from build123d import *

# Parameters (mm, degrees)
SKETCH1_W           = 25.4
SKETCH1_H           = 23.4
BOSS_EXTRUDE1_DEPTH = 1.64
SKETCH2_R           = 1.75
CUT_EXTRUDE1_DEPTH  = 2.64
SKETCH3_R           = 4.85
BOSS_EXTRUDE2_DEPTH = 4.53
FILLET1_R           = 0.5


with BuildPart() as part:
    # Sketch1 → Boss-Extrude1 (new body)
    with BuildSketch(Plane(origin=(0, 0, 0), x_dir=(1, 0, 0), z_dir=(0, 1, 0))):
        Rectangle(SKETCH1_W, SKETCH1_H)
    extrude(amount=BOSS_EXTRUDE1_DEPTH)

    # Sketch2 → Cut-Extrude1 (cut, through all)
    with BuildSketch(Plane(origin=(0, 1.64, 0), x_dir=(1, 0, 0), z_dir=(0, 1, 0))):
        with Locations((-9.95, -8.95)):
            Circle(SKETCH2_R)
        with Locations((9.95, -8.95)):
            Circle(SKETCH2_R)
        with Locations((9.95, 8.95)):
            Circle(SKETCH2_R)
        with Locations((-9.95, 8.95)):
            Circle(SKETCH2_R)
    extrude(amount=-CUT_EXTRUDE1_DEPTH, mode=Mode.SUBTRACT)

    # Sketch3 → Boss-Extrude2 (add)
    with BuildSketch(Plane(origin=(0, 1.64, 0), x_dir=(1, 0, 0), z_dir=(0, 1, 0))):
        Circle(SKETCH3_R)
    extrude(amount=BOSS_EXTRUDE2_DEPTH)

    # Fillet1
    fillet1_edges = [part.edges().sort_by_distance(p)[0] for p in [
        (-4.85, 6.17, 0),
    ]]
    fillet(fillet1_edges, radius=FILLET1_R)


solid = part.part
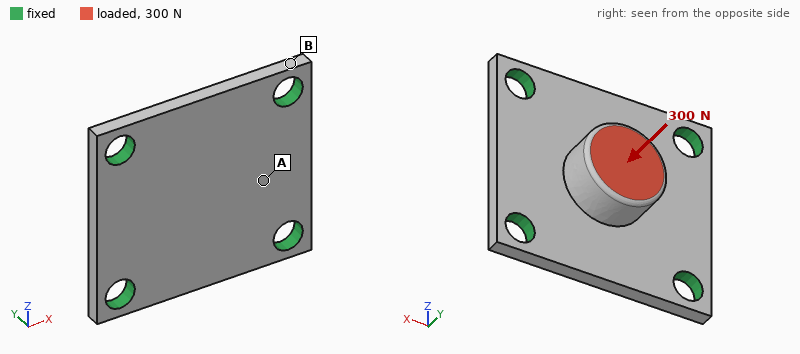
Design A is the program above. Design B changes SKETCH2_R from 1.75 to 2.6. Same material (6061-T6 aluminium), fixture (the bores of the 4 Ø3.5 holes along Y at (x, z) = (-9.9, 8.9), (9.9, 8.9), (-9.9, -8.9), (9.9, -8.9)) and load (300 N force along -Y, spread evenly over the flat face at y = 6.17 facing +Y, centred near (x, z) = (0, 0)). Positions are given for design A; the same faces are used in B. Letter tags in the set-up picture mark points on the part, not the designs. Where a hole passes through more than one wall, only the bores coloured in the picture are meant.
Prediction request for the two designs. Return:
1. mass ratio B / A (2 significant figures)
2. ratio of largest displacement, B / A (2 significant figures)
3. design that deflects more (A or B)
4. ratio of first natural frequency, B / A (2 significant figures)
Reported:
0.94
0.73
A
1.2
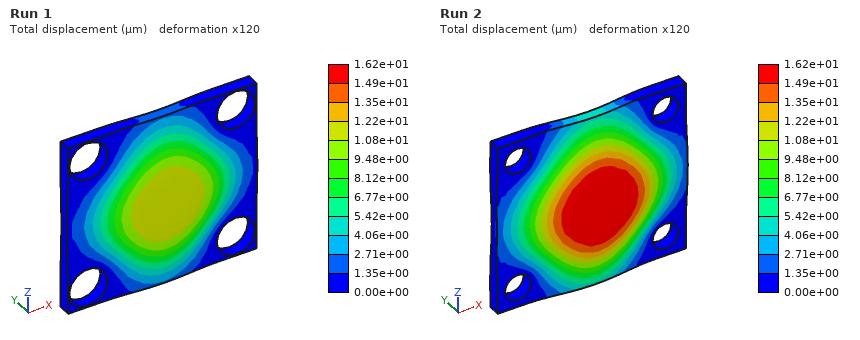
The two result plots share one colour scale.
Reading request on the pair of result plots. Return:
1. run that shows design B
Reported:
Run 1
